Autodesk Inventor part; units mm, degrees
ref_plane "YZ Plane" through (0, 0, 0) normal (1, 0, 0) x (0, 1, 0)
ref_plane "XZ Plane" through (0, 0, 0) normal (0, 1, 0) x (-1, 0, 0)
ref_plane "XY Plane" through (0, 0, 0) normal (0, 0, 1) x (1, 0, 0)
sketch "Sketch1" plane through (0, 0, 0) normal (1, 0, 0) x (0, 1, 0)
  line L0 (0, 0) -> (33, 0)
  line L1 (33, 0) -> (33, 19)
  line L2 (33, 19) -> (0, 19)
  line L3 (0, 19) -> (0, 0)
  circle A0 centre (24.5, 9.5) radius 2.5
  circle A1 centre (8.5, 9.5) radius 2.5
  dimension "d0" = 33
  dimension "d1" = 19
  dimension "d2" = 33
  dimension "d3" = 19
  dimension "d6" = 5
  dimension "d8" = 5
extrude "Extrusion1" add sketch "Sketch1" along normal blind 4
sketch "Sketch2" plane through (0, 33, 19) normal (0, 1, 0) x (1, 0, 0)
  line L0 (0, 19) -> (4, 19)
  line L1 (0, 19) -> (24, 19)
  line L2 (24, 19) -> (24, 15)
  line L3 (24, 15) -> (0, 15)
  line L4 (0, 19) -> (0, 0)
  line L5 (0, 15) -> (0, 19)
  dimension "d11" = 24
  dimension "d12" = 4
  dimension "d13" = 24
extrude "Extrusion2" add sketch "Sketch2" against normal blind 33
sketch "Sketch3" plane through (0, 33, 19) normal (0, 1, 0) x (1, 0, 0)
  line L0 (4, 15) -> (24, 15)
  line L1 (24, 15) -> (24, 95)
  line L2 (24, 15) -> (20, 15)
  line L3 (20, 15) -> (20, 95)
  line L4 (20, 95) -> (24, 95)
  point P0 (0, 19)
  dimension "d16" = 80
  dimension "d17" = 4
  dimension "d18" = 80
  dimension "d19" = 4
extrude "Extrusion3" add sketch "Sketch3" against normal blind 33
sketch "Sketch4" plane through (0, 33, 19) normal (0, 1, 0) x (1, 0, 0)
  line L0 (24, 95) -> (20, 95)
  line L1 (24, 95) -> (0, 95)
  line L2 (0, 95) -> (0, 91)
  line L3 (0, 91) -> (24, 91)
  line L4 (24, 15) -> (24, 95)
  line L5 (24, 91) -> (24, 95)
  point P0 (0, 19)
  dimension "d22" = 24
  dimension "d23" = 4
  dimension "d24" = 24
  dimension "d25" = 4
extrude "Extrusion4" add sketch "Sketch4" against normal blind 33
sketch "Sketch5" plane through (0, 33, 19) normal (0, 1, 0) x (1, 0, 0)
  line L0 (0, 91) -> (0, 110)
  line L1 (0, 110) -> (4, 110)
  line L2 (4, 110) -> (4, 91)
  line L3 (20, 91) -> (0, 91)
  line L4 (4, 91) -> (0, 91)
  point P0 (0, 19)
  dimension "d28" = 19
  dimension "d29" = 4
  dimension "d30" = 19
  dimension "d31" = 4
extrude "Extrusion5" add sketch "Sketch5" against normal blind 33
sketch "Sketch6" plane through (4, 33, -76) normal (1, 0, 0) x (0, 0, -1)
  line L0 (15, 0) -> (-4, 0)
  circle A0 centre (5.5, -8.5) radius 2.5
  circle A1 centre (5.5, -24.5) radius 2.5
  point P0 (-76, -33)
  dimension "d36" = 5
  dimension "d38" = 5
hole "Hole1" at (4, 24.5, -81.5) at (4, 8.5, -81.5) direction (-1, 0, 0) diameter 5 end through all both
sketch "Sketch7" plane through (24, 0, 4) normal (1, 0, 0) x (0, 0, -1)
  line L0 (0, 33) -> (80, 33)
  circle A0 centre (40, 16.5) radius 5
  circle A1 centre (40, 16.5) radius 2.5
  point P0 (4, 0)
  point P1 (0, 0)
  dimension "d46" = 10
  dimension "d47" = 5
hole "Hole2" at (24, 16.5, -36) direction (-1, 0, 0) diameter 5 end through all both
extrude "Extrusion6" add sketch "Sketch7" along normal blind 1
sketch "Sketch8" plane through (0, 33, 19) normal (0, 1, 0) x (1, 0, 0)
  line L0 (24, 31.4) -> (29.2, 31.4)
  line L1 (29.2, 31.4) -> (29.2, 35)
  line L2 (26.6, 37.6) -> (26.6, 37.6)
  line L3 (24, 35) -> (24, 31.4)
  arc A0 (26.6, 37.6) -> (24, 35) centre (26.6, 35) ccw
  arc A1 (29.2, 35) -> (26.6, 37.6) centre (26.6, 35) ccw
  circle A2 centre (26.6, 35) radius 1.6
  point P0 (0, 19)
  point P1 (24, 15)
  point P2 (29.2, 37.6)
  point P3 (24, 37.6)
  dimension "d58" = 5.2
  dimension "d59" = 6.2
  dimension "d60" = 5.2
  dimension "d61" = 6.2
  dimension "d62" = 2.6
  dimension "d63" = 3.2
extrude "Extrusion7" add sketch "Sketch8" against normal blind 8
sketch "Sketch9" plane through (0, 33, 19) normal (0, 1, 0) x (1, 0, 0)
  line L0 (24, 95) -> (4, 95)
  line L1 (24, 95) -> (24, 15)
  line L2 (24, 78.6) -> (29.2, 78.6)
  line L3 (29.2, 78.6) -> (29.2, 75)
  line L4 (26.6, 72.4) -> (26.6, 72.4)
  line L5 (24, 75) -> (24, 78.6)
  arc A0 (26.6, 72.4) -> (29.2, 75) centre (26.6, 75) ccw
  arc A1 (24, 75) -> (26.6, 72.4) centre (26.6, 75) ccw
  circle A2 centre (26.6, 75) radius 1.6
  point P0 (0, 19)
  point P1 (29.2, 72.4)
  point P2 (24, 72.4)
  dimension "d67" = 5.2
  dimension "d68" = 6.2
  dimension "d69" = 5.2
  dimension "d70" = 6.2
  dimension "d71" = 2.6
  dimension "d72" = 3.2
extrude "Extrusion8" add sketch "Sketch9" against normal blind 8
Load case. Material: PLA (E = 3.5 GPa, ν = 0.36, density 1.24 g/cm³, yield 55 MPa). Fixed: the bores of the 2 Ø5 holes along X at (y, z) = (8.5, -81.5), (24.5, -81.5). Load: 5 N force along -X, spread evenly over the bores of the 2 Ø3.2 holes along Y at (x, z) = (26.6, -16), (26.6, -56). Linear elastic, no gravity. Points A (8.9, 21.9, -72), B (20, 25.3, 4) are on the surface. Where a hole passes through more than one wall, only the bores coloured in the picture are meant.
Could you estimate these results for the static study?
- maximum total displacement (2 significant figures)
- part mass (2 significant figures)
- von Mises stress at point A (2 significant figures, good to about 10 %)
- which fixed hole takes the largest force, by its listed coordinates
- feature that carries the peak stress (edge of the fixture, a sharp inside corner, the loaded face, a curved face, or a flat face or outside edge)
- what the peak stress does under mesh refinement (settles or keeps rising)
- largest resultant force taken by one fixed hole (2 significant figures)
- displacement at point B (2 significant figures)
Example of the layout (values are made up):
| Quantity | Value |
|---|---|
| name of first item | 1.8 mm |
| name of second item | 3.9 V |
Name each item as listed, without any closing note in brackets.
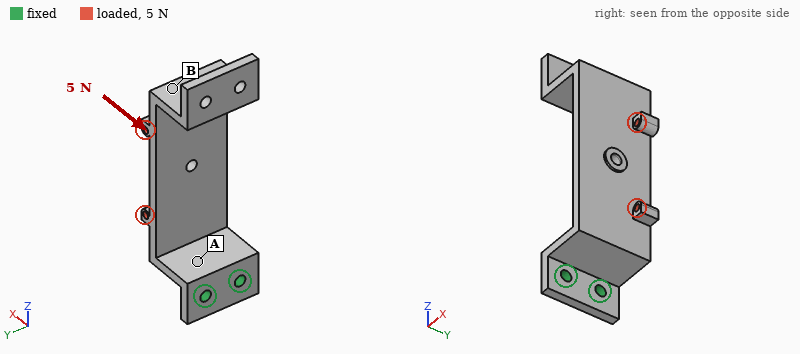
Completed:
| Quantity | Value |
|---|---|
| maximum total displacement | 1.2 mm |
| part mass | 25 g |
| von Mises stress at point A | 2.0 MPa |
| which fixed hole takes the largest force, by its listed coordinates | (24.5, -81.5) |
| feature that carries the peak stress | edge of the fixture |
| what the peak stress does under mesh refinement | keeps rising |
| largest resultant force taken by one fixed hole | 5.6 N |
| displacement at point B | 0.98 mm |
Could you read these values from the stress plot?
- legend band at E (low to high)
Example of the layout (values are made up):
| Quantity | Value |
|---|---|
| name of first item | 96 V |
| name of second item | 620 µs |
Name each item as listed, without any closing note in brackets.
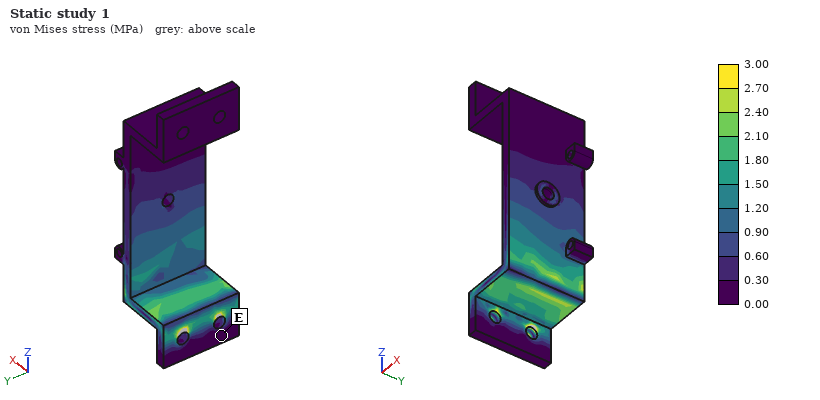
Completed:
| Quantity | Value |
|---|---|
| legend band at E | 0.00 to 0.30 MPa |
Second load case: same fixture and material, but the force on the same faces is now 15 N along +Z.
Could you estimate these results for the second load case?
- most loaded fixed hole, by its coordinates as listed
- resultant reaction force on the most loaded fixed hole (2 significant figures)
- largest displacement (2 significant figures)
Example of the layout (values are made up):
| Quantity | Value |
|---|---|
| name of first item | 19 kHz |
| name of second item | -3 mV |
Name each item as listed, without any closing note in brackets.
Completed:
| Quantity | Value |
|---|---|
| most loaded fixed hole, by its coordinates as listed | (24.5, -81.5) |
| resultant reaction force on the most loaded fixed hole | 17 N |
| largest displacement | 1.2 mm |
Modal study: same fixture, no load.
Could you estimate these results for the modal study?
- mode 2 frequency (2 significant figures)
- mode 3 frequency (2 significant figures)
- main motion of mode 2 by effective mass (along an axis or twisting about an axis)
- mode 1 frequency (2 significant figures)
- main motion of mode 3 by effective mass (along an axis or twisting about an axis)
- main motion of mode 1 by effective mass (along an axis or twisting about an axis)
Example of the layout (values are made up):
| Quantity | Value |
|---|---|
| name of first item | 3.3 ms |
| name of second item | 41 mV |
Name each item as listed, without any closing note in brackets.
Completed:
| Quantity | Value |
|---|---|
| mode 2 frequency | 160 Hz |
| mode 3 frequency | 360 Hz |
| main motion of mode 2 by effective mass | along Y |
| mode 1 frequency | 75 Hz |
| main motion of mode 3 by effective mass | along Z |
| main motion of mode 1 by effective mass | along X |
